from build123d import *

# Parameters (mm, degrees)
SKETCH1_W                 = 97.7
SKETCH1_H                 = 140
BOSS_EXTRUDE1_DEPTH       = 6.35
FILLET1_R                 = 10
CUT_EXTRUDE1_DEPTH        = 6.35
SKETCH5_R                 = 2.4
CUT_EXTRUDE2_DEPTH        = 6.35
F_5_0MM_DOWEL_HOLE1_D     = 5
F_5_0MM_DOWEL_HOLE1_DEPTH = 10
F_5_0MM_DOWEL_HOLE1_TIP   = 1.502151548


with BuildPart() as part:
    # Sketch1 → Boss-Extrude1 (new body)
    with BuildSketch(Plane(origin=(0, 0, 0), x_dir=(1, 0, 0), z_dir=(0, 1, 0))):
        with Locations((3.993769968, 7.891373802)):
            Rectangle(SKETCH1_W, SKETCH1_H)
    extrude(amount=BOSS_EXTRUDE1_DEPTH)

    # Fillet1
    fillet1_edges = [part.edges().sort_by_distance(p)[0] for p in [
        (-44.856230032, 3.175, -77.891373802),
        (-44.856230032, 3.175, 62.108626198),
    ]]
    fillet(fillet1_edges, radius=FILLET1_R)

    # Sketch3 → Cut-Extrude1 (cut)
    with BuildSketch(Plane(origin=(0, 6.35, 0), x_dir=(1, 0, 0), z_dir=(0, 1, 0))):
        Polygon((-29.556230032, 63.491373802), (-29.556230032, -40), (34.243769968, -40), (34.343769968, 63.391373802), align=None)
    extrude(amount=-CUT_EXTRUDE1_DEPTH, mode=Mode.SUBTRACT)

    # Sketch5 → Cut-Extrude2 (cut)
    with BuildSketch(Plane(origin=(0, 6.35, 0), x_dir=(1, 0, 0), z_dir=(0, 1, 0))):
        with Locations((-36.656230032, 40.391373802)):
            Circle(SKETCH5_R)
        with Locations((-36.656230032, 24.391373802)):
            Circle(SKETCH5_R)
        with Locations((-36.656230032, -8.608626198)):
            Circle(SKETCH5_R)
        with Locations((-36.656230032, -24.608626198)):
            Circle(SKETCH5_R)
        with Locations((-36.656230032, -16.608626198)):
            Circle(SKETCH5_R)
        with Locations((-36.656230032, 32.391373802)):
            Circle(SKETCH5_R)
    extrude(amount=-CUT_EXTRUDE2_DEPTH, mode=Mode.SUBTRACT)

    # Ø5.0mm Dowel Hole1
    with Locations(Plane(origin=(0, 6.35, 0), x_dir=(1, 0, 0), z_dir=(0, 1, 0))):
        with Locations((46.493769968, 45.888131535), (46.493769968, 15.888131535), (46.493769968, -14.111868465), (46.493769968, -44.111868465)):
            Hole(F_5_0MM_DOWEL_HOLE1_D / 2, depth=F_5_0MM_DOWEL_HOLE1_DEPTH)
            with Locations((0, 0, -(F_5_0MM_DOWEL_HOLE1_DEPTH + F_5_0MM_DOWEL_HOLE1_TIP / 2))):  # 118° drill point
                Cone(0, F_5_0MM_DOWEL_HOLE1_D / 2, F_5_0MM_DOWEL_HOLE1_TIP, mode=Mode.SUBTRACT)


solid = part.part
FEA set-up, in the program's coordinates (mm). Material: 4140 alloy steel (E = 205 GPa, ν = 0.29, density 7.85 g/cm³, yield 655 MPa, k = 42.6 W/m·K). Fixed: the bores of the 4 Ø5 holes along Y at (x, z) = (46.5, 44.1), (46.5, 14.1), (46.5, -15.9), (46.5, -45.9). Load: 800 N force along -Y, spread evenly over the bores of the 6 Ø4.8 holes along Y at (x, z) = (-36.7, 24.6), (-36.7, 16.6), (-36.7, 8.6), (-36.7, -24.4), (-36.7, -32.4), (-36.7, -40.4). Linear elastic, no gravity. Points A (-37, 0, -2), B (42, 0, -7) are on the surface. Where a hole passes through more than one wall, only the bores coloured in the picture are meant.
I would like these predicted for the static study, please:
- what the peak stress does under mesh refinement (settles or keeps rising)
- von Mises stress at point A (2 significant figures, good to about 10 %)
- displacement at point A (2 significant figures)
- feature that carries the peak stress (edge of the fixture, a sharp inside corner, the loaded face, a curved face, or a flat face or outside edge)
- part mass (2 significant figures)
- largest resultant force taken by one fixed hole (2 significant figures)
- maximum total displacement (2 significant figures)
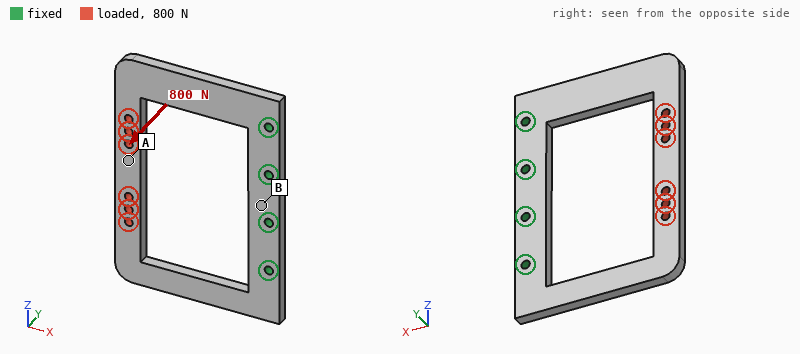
keeps rising
69 MPa
1.2 mm
edge of the fixture
340 g
510 N
1.4 mm
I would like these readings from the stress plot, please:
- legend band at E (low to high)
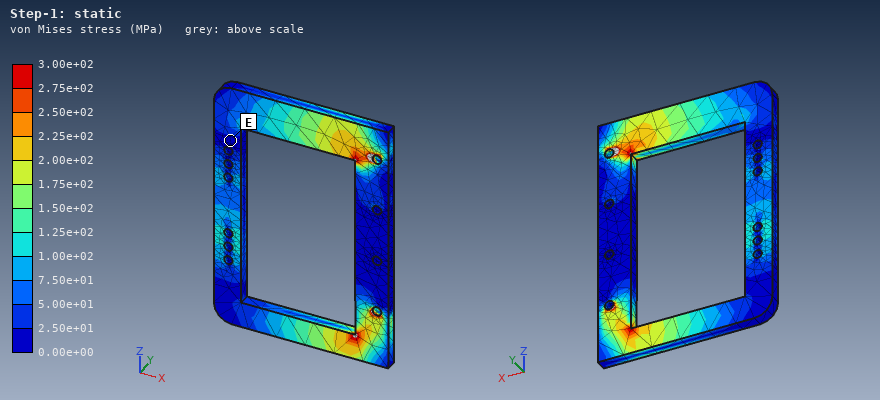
0.00e+00 to 2.50e+01 MPa
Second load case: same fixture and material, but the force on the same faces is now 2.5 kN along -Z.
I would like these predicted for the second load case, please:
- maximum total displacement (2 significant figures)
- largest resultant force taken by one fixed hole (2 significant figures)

0.25 mm
3.4 kN
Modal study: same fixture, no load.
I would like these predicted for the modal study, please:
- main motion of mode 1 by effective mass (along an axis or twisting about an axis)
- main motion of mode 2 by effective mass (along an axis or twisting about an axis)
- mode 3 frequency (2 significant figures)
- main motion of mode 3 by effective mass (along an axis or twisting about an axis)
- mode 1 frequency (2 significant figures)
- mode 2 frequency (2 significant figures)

along Y
twisting about X
1400 Hz
along Z
380 Hz
720 Hz
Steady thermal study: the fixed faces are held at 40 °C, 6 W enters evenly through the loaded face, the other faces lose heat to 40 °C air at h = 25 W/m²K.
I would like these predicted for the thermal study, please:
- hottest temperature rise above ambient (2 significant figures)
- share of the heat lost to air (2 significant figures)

31 K
78 %
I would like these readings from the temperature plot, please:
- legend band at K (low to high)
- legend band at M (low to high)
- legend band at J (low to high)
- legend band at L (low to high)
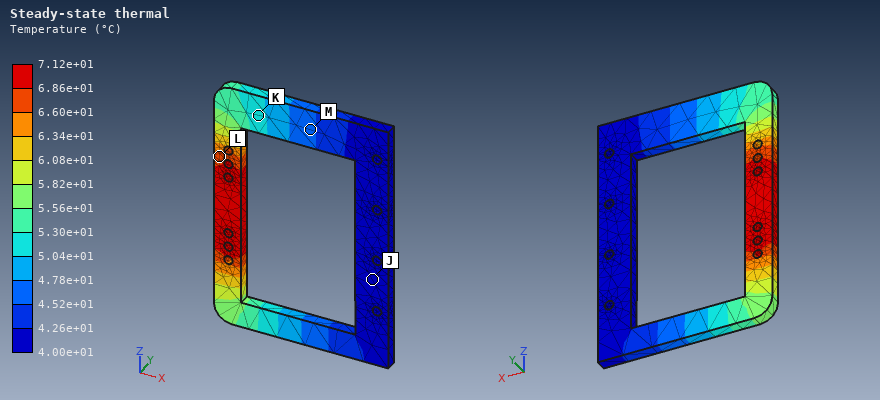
5.04e+01 to 5.30e+01 °C
4.52e+01 to 4.78e+01 °C
4.00e+01 to 4.26e+01 °C
6.60e+01 to 6.86e+01 °C
